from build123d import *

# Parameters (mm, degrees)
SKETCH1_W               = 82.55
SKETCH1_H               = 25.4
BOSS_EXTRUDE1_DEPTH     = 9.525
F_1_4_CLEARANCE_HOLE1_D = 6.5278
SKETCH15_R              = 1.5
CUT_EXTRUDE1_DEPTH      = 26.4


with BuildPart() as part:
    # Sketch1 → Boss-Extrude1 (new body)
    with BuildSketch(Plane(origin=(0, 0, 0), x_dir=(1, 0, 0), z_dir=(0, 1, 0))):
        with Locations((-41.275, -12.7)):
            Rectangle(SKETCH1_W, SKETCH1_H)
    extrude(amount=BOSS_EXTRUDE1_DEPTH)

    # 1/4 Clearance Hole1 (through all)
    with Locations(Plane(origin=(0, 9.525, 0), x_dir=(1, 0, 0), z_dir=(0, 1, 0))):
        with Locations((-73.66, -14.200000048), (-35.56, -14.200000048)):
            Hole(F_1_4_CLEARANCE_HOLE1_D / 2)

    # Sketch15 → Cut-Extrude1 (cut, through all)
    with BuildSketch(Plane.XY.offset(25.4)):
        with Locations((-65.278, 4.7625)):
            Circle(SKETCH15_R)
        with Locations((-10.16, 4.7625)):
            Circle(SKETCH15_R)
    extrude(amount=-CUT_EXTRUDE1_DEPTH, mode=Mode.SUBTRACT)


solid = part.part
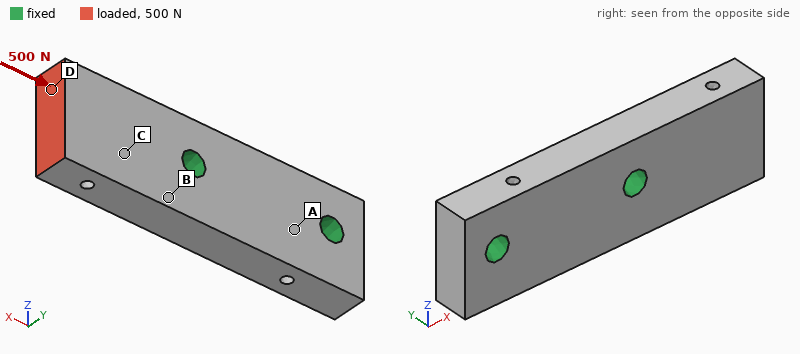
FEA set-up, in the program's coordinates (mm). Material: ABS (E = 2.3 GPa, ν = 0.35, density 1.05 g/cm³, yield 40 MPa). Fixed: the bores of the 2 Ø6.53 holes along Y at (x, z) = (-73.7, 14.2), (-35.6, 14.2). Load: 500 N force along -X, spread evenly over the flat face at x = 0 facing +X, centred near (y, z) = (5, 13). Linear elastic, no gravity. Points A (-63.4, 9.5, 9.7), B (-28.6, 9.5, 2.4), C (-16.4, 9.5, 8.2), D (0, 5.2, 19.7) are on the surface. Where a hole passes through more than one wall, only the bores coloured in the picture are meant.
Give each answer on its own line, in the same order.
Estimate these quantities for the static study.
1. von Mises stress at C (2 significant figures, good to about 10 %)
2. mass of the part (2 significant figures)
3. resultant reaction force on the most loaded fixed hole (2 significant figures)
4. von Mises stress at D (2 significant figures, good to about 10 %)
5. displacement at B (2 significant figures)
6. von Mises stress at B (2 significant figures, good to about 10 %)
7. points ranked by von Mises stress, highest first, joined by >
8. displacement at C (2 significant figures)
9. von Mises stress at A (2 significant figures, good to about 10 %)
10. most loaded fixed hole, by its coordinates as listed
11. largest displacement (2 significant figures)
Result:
2.4 MPa
20 g
450 N
2.0 MPa
15 µm
1.5 MPa
C > D > B > A
23 µm
0.38 MPa
(-35.6, 14.2)
44 µm
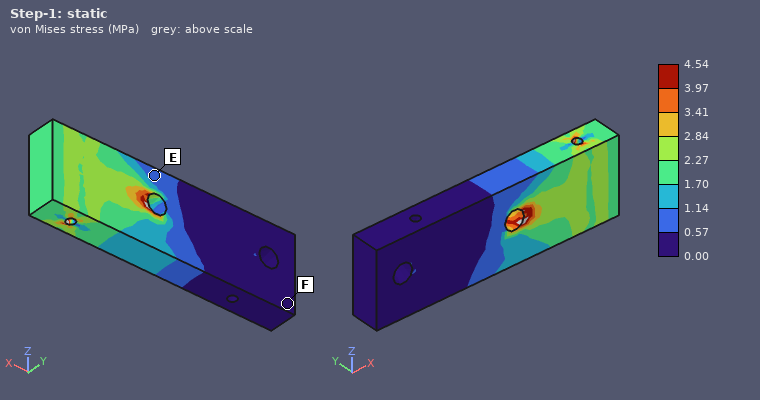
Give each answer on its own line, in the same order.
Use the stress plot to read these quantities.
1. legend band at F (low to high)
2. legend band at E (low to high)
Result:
0.00 to 0.57 MPa
0.57 to 1.14 MPa
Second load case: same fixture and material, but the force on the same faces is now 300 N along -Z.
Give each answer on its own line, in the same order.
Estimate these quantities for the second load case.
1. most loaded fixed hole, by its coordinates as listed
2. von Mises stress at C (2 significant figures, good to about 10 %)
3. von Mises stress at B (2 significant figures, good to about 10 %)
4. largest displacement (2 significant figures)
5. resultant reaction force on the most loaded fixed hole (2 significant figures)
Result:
(-35.6, 14.2)
3.4 MPa
6.5 MPa
0.37 mm
470 N
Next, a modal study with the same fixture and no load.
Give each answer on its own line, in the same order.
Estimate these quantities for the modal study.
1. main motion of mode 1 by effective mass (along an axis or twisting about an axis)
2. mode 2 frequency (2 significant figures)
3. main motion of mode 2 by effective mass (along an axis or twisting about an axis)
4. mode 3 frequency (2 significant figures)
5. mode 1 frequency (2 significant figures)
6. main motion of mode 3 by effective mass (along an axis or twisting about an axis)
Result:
along Y
2800 Hz
along Z
4000 Hz
1800 Hz
twisting about X
